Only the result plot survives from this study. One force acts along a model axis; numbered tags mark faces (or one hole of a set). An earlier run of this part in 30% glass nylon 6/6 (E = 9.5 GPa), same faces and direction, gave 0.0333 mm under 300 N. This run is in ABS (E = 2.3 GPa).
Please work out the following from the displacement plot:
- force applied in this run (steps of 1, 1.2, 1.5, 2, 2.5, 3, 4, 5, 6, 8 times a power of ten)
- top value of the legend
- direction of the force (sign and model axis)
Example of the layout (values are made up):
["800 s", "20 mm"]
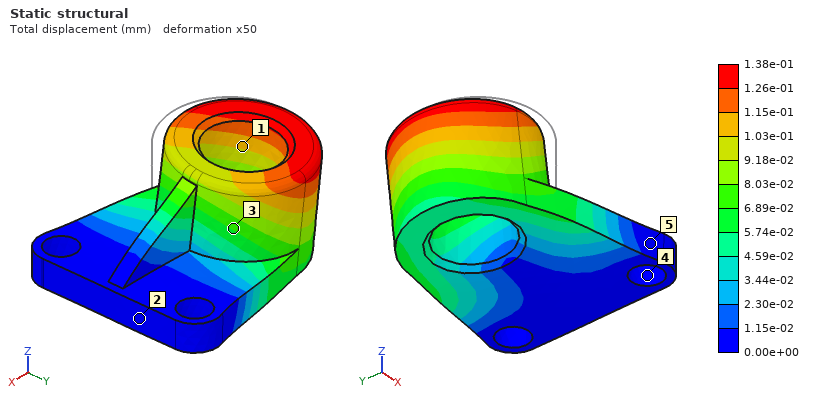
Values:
["300 N", "1.38e-01 mm", "+Y"]
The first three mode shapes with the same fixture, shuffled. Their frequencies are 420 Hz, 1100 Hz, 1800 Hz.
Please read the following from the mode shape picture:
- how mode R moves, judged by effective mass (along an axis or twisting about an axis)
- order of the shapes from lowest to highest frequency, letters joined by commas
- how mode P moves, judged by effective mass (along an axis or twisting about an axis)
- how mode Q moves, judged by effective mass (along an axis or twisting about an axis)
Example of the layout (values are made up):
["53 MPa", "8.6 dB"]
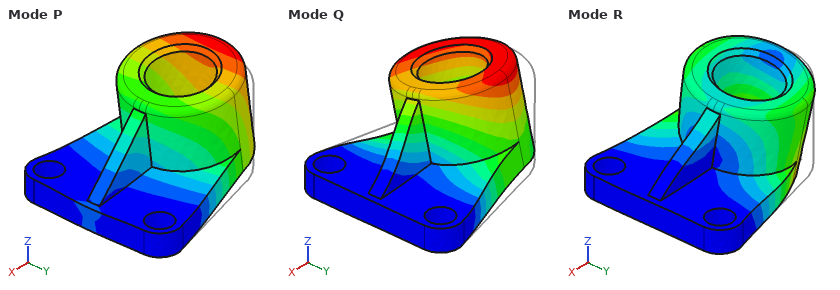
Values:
["along Y", "P, Q, R", "along Z", "along Y"]
